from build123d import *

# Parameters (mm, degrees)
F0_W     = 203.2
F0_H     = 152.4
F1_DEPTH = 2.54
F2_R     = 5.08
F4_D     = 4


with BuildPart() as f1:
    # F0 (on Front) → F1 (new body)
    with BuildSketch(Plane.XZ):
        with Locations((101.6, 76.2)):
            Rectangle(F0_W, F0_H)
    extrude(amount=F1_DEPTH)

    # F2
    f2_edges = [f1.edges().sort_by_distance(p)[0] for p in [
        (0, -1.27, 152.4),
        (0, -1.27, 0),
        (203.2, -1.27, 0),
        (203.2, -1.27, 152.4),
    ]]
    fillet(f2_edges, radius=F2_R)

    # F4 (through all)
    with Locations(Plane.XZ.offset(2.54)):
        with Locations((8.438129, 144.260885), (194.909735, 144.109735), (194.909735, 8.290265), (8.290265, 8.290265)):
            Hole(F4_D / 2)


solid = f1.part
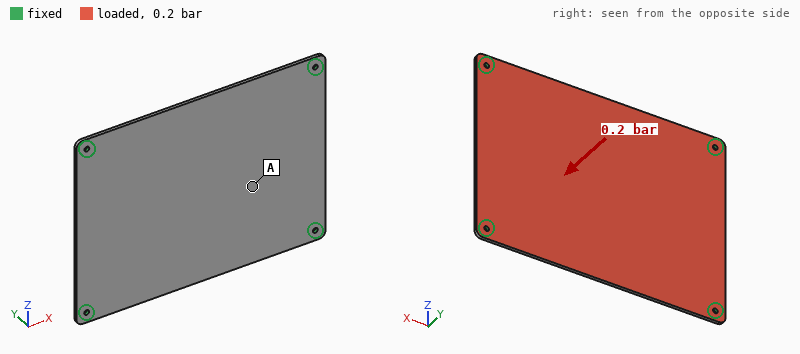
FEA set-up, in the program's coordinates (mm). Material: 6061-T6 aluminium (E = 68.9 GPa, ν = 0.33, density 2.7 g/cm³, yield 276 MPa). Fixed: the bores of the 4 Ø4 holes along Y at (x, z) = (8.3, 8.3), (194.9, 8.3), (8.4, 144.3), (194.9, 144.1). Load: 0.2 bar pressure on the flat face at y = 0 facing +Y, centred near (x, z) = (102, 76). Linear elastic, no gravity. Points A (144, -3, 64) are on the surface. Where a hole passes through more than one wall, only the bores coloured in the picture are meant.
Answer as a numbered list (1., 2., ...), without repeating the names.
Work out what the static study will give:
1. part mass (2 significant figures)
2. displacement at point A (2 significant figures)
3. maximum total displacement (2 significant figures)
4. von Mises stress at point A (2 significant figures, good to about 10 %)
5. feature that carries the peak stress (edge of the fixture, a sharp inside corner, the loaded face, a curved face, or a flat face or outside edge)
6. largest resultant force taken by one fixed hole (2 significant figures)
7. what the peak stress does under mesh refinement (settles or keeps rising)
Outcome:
1. 210 g
2. 1.0 mm
3. 1.3 mm
4. 23 MPa
5. edge of the fixture
6. 150 N
7. keeps rising
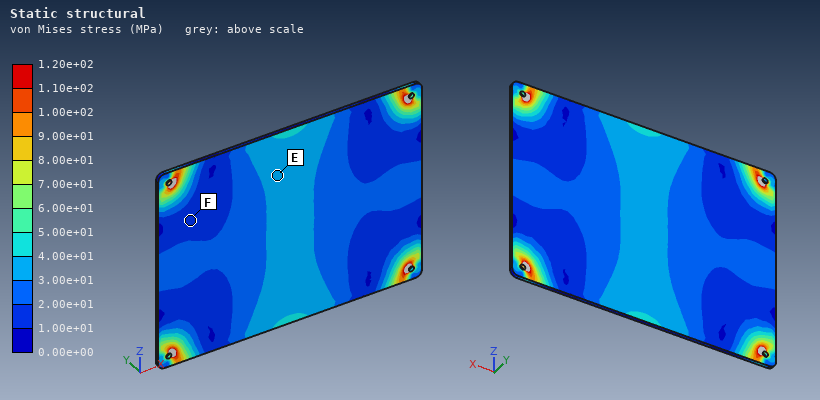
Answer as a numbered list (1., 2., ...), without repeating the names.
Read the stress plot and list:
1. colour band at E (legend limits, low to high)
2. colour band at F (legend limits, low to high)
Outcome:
1. 3.00e+01 to 4.00e+01 MPa
2. 1.00e+01 to 2.00e+01 MPa
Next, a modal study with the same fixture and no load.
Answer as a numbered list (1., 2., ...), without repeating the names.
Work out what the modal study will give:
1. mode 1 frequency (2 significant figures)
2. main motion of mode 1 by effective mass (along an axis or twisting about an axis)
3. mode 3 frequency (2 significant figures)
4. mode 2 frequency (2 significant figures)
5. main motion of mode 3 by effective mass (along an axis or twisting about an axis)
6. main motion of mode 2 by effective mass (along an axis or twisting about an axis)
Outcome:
1. 280 Hz
2. along Y
3. 640 Hz
4. 470 Hz
5. twisting about Z
6. twisting about X
